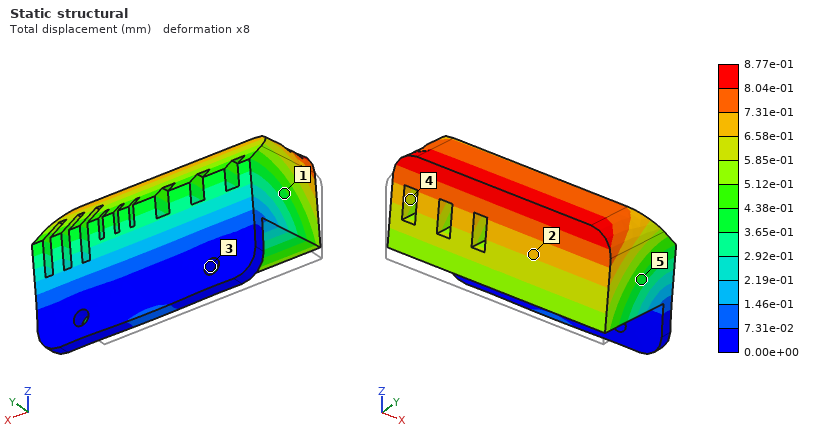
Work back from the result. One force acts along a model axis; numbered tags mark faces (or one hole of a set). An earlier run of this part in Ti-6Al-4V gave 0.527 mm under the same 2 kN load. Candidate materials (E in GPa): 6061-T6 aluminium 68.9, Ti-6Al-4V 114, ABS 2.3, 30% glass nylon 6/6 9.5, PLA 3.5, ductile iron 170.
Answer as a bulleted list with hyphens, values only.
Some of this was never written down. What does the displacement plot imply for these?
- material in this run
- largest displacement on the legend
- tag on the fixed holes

- 6061-T6 aluminium
- 8.77e-01 mm
- 3
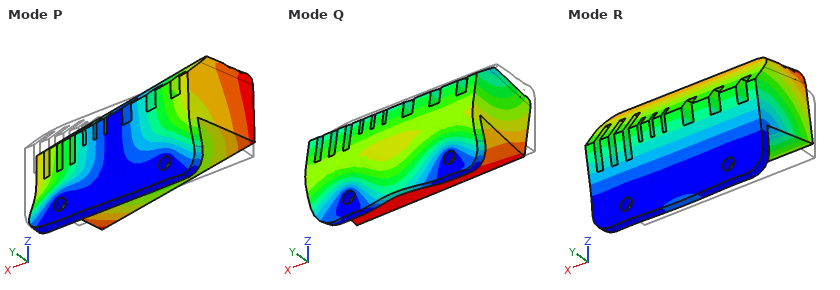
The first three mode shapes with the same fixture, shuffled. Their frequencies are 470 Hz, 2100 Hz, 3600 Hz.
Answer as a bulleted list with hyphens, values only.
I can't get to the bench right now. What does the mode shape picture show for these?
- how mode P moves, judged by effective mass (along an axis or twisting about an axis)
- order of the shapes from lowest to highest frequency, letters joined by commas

- along X
- R, P, Q
